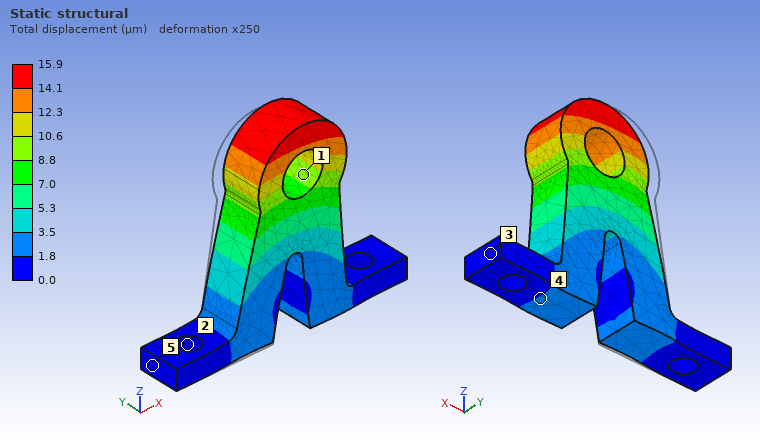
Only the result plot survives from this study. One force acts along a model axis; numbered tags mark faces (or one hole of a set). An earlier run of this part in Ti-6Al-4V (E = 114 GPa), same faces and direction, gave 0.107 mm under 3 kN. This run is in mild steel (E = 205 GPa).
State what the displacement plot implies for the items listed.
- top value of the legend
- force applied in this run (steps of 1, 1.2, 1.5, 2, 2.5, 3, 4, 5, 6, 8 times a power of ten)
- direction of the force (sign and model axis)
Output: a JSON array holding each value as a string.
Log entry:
["15.9 µm", "800 N", "+X"]
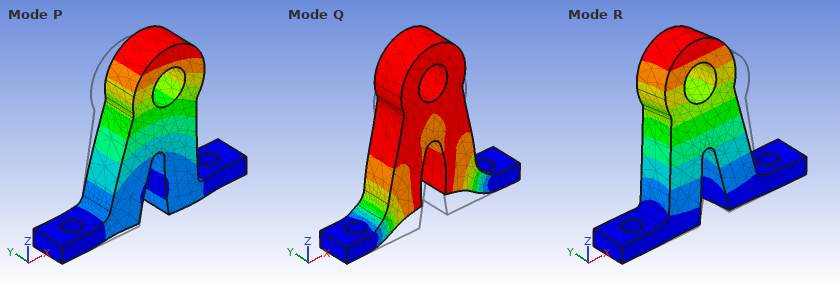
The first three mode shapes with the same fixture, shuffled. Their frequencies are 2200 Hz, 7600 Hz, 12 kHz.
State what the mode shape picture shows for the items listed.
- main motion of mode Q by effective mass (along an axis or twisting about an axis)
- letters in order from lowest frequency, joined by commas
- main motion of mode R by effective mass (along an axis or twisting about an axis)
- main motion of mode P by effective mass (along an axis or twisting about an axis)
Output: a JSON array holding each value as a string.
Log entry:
["along Z", "R, P, Q", "along Y", "along X"]
